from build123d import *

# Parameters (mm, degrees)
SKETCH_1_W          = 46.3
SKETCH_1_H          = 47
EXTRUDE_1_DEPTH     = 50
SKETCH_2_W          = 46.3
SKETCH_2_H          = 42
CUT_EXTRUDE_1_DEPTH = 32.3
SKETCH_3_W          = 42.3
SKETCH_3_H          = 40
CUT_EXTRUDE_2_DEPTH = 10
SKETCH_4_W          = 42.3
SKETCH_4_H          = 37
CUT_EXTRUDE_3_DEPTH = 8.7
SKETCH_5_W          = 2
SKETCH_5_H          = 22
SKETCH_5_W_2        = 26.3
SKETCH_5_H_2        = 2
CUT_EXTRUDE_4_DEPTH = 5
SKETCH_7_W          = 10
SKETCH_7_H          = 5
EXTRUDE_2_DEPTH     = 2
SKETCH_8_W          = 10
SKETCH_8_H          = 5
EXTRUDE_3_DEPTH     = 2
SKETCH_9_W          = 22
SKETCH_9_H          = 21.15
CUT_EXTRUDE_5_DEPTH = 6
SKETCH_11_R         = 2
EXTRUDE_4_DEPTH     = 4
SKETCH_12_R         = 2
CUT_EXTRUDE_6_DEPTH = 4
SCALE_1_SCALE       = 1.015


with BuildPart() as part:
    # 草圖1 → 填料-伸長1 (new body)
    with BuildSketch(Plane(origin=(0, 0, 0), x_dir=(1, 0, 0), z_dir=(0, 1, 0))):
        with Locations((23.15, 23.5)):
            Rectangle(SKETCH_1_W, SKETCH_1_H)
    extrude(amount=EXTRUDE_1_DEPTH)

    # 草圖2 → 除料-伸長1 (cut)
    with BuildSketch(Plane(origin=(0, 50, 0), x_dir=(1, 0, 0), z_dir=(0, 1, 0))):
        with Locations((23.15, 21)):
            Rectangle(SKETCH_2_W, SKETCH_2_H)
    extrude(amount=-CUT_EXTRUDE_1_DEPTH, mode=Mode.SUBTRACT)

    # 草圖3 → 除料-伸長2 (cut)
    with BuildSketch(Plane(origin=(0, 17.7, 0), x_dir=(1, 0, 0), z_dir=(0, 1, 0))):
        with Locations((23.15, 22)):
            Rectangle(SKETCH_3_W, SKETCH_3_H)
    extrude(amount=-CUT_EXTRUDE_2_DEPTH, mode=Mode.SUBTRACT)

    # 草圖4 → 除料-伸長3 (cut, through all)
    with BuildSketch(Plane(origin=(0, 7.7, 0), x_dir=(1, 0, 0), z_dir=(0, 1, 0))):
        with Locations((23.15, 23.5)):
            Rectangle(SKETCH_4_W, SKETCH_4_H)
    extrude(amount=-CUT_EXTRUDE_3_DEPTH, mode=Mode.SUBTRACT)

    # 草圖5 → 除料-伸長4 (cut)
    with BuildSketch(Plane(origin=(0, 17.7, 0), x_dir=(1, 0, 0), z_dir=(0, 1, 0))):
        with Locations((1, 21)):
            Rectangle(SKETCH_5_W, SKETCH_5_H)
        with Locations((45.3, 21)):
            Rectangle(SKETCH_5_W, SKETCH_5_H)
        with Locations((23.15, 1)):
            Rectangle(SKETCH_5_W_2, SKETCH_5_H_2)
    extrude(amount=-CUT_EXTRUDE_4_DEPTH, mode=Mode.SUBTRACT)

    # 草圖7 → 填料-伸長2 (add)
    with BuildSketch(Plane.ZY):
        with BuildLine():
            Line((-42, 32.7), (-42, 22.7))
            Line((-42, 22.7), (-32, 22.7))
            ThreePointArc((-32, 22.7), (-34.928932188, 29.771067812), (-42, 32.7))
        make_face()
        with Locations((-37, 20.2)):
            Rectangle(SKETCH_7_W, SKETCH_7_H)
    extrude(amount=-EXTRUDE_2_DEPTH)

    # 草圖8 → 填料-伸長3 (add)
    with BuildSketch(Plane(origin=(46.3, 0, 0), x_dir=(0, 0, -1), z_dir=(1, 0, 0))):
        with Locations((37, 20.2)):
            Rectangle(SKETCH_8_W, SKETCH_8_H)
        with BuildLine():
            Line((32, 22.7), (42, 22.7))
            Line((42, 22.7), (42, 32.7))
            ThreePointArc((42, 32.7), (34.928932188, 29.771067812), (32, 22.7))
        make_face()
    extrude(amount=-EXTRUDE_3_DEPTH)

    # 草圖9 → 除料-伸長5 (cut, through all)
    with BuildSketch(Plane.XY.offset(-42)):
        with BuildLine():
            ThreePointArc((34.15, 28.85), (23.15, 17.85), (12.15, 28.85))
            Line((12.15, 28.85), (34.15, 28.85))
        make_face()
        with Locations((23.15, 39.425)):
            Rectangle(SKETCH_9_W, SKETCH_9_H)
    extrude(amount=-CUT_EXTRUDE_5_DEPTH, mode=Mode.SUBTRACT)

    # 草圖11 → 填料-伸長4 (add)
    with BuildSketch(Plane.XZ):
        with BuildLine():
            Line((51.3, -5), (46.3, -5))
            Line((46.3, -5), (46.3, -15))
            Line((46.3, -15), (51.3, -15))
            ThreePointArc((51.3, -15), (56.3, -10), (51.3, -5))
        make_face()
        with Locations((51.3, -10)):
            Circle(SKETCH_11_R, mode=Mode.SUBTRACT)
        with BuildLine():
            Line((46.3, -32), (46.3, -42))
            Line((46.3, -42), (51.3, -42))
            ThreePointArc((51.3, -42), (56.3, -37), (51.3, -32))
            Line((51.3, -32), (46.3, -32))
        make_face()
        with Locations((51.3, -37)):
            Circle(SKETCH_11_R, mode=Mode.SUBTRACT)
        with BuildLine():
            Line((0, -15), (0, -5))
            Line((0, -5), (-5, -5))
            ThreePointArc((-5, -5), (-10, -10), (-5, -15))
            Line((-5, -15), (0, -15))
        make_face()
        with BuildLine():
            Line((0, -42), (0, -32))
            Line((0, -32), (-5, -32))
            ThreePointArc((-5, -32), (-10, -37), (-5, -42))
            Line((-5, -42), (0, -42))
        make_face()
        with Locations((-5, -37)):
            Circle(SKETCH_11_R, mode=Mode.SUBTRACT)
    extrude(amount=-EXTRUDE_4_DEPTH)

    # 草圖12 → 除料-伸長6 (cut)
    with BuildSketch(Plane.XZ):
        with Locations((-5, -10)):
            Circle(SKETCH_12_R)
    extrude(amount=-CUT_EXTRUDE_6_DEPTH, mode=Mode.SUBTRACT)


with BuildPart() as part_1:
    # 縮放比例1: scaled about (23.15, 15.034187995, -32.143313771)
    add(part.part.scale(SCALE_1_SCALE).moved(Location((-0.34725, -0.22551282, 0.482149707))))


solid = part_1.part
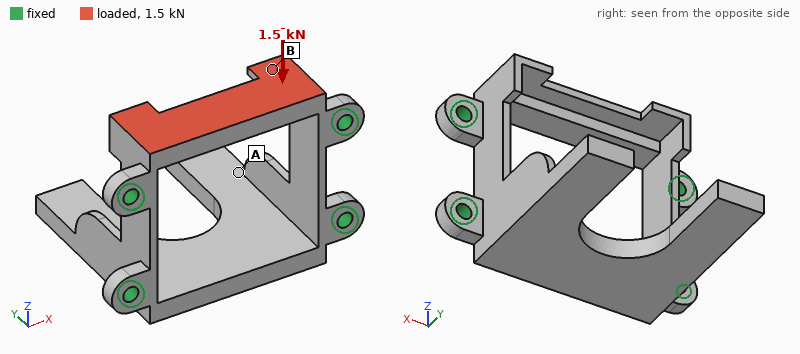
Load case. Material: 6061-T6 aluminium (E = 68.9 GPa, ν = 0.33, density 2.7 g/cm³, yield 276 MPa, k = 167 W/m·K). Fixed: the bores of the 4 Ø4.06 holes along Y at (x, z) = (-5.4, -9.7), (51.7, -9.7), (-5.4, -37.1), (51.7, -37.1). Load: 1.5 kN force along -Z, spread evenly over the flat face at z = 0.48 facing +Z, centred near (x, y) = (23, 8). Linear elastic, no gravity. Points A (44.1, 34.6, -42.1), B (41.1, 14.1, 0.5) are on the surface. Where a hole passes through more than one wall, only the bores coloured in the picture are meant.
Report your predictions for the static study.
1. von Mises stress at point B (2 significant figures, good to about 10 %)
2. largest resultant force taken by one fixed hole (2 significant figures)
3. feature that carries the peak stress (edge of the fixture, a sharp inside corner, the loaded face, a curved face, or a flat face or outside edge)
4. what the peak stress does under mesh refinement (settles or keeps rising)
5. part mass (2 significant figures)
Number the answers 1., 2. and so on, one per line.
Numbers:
1. 28 MPa
2. 910 N
3. a sharp inside corner
4. keeps rising
5. 42 g
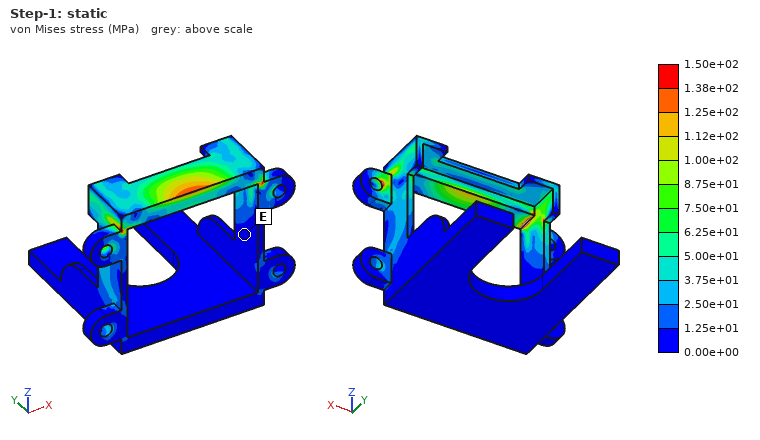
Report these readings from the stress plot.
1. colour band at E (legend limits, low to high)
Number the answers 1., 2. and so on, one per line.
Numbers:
1. 0.00e+00 to 1.25e+01 MPa
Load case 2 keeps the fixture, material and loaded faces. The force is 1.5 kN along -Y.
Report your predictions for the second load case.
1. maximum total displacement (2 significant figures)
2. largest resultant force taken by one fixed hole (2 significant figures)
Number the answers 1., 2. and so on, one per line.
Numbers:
1. 0.13 mm
2. 1.0 kN
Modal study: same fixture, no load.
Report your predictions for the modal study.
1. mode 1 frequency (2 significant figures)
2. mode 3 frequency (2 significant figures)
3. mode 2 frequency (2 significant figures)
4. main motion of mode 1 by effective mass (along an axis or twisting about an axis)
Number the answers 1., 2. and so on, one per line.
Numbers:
1. 2700 Hz
2. 6100 Hz
3. 3300 Hz
4. along Z
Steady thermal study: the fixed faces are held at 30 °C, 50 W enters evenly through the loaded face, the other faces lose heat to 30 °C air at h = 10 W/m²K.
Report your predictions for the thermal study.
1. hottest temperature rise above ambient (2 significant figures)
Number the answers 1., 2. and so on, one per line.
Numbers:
1. 71 K
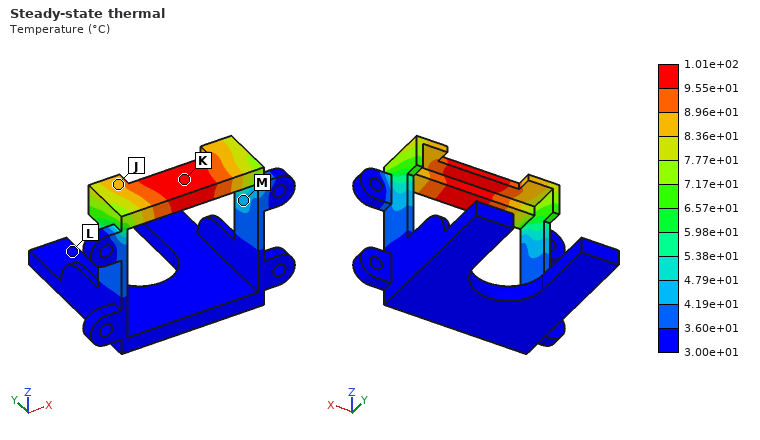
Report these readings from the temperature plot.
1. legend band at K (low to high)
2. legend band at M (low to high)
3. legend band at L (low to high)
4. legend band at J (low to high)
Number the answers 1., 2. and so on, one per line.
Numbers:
1. 9.55e+01 to 1.01e+02 °C
2. 4.19e+01 to 4.79e+01 °C
3. 3.00e+01 to 3.60e+01 °C
4. 8.36e+01 to 8.96e+01 °C
